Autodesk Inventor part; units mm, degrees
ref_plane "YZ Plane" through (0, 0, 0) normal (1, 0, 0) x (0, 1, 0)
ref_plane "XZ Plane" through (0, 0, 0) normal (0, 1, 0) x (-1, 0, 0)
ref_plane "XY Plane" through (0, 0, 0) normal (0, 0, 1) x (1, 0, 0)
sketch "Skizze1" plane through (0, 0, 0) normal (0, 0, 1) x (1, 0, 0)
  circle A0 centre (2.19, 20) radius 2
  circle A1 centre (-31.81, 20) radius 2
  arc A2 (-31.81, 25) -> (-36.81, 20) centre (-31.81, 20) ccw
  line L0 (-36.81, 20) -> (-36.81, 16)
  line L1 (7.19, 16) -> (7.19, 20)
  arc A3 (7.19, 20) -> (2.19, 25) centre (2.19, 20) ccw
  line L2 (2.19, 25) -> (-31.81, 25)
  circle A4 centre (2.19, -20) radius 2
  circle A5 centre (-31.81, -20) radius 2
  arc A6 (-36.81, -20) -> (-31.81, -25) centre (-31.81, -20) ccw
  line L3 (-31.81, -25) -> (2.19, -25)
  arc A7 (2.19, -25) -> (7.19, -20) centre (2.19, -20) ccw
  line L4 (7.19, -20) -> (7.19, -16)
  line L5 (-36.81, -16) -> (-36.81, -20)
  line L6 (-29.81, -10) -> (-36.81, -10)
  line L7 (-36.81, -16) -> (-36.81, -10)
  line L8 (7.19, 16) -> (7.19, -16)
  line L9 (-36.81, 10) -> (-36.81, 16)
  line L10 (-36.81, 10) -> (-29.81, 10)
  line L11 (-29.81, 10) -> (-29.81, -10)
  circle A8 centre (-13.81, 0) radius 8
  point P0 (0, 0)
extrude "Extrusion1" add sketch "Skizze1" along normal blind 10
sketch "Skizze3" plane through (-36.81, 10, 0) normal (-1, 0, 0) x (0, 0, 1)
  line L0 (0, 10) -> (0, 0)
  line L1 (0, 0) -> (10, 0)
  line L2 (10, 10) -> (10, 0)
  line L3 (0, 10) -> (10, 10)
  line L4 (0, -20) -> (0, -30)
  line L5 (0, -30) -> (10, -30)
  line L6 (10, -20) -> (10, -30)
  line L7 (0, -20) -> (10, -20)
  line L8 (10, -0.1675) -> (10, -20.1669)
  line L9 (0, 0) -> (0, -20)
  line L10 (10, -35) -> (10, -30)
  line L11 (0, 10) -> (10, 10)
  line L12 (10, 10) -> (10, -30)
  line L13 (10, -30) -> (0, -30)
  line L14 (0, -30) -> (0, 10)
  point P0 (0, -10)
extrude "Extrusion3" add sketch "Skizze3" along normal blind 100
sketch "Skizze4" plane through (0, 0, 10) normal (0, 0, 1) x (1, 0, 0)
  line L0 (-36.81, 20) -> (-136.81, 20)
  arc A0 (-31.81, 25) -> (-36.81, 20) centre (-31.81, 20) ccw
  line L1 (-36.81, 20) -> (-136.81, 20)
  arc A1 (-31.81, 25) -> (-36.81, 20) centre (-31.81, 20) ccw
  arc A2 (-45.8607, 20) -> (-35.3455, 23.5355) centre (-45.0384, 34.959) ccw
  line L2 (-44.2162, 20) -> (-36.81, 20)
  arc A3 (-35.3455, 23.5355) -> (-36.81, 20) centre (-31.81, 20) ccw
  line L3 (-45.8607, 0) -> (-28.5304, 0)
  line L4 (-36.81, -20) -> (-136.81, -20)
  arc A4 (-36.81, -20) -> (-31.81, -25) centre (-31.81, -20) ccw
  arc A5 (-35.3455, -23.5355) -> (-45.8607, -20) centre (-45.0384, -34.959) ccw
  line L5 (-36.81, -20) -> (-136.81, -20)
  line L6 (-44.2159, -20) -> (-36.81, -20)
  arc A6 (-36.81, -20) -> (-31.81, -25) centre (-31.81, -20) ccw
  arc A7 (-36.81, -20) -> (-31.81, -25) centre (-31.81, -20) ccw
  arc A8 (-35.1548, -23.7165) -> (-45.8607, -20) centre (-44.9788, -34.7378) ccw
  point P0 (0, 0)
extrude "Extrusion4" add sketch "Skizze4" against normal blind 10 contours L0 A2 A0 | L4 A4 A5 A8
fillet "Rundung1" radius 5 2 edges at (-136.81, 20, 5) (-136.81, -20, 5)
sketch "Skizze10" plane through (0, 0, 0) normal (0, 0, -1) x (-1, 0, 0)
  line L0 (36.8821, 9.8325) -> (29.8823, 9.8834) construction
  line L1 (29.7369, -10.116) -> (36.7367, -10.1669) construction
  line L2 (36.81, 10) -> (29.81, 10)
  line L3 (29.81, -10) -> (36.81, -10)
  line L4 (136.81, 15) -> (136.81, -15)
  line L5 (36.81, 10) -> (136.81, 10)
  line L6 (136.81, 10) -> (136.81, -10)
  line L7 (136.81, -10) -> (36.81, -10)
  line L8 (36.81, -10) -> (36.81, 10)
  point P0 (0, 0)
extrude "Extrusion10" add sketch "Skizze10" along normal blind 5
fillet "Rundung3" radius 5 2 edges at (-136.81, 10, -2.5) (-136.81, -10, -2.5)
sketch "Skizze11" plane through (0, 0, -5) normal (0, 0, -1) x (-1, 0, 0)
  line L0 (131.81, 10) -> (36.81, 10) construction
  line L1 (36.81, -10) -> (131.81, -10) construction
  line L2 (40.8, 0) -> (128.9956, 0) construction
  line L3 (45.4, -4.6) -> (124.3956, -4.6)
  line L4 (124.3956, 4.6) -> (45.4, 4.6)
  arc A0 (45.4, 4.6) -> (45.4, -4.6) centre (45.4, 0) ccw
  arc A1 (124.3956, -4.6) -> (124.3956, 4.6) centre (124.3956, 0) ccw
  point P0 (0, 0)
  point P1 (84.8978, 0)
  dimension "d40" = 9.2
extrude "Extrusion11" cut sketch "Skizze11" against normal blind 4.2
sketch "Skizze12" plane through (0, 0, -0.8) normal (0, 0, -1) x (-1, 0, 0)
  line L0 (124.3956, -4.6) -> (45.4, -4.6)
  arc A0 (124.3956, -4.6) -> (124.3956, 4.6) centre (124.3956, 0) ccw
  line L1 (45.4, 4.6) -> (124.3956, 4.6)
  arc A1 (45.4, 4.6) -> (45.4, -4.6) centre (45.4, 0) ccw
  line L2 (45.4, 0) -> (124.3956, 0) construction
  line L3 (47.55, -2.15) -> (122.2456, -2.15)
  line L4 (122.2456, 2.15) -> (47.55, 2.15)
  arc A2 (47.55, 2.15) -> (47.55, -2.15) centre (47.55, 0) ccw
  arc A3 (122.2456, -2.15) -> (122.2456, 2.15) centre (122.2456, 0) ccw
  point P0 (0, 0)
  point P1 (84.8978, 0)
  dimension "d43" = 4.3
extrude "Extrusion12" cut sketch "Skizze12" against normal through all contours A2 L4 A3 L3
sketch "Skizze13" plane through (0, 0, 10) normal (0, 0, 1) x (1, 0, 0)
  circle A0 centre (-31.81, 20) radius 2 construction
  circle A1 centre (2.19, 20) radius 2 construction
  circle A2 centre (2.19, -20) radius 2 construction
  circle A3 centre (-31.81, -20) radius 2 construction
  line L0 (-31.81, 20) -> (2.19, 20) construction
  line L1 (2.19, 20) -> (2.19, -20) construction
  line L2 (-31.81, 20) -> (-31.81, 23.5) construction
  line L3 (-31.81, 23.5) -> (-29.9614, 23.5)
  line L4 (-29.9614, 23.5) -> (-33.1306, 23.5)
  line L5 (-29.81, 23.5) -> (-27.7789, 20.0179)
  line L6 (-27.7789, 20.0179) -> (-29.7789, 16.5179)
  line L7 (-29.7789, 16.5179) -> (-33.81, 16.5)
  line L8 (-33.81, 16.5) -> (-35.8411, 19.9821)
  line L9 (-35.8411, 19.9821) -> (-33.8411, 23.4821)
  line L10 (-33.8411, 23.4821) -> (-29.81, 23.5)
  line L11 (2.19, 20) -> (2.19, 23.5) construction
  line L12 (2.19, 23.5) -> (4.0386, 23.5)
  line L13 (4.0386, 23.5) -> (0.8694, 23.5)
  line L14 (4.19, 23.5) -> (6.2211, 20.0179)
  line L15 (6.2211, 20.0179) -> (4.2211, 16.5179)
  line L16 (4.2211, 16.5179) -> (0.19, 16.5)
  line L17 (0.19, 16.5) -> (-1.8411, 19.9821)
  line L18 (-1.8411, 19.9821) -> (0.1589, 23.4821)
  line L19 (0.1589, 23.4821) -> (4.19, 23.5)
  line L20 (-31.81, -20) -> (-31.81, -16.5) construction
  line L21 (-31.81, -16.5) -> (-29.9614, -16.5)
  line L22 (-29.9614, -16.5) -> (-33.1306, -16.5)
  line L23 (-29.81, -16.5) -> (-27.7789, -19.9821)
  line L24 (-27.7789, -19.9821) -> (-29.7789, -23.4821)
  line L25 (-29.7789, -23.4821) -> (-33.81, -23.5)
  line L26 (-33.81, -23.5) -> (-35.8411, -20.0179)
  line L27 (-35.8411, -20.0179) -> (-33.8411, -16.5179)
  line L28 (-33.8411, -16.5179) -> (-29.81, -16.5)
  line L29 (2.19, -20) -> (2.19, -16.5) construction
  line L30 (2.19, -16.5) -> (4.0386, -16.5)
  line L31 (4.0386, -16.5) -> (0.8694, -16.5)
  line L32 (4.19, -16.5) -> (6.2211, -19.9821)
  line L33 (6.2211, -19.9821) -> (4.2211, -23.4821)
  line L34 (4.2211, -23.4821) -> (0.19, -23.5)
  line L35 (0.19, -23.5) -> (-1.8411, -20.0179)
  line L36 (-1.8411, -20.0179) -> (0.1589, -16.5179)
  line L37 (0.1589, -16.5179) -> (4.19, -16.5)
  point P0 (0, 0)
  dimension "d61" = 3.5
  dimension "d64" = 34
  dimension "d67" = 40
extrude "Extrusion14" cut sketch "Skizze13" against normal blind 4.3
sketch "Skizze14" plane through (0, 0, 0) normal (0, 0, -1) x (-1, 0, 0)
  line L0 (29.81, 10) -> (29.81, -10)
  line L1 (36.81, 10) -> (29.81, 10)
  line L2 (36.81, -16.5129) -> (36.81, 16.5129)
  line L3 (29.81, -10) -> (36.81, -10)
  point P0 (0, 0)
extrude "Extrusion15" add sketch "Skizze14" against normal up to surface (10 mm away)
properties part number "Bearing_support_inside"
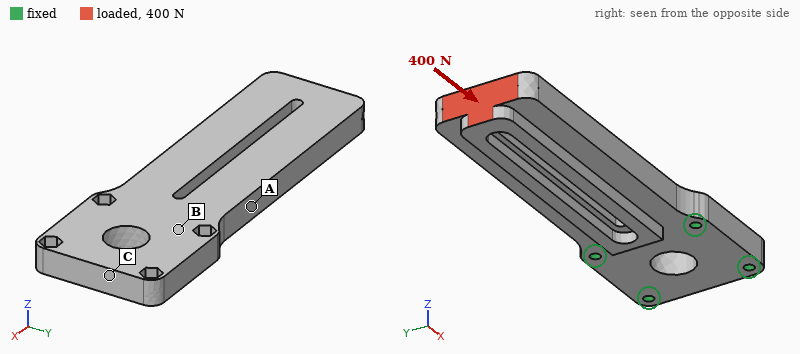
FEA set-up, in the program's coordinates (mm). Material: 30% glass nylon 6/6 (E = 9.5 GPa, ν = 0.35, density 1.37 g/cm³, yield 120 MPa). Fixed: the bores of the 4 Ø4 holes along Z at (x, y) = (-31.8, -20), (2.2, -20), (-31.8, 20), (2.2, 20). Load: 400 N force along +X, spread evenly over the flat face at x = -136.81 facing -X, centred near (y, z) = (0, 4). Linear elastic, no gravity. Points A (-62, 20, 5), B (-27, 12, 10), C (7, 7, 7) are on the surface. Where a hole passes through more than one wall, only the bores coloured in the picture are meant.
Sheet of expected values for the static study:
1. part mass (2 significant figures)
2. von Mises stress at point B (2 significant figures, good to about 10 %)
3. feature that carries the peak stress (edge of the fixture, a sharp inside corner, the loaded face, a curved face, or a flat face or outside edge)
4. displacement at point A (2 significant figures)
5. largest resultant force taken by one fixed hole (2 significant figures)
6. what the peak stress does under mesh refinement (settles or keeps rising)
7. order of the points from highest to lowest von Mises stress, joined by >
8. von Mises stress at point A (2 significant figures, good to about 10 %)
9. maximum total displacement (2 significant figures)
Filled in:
85 g
0.70 MPa
edge of the fixture
4.9 µm
160 N
keeps rising
A > B > C
1.2 MPa
16 µm
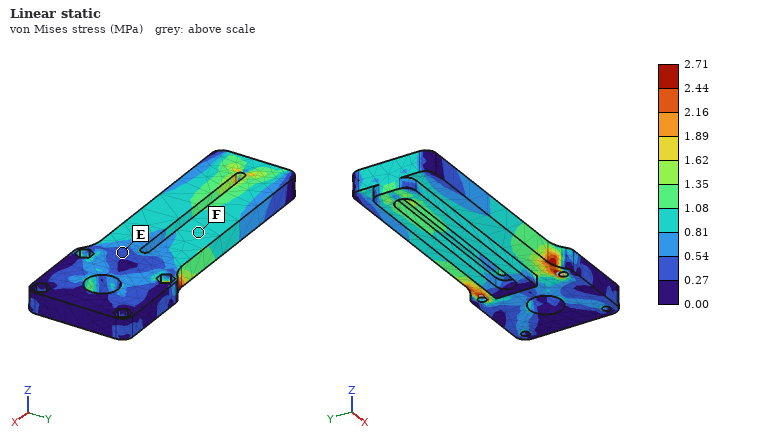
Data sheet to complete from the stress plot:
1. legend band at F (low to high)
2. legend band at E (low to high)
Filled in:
0.81 to 1.08 MPa
0.27 to 0.54 MPa
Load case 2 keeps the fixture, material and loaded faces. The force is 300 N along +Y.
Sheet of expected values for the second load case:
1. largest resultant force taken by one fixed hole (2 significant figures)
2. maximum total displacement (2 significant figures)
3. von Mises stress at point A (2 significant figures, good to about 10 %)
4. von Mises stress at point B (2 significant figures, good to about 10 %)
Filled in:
720 N
0.40 mm
12 MPa
3.3 MPa
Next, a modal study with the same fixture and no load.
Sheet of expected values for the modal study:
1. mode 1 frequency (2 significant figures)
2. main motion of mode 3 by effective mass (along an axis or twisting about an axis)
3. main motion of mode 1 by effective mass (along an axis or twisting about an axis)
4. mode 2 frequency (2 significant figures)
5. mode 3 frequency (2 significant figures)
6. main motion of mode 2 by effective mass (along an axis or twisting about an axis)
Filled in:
360 Hz
twisting about X
along Z
990 Hz
1600 Hz
along Y
